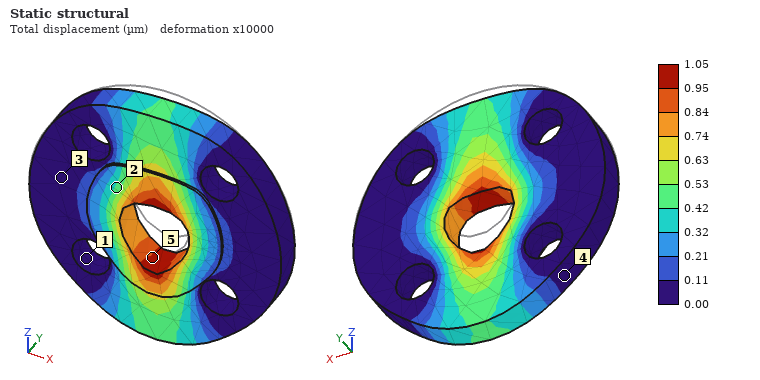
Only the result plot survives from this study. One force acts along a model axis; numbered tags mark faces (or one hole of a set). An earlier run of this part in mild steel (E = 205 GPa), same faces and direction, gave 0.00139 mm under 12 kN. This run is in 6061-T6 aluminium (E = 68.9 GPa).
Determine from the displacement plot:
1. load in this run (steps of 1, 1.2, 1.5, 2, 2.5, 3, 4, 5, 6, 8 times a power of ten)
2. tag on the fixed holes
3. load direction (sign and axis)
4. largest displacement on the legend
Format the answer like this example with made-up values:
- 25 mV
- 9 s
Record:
- 3 kN
- 1
- -Z
- 1.05 µm
